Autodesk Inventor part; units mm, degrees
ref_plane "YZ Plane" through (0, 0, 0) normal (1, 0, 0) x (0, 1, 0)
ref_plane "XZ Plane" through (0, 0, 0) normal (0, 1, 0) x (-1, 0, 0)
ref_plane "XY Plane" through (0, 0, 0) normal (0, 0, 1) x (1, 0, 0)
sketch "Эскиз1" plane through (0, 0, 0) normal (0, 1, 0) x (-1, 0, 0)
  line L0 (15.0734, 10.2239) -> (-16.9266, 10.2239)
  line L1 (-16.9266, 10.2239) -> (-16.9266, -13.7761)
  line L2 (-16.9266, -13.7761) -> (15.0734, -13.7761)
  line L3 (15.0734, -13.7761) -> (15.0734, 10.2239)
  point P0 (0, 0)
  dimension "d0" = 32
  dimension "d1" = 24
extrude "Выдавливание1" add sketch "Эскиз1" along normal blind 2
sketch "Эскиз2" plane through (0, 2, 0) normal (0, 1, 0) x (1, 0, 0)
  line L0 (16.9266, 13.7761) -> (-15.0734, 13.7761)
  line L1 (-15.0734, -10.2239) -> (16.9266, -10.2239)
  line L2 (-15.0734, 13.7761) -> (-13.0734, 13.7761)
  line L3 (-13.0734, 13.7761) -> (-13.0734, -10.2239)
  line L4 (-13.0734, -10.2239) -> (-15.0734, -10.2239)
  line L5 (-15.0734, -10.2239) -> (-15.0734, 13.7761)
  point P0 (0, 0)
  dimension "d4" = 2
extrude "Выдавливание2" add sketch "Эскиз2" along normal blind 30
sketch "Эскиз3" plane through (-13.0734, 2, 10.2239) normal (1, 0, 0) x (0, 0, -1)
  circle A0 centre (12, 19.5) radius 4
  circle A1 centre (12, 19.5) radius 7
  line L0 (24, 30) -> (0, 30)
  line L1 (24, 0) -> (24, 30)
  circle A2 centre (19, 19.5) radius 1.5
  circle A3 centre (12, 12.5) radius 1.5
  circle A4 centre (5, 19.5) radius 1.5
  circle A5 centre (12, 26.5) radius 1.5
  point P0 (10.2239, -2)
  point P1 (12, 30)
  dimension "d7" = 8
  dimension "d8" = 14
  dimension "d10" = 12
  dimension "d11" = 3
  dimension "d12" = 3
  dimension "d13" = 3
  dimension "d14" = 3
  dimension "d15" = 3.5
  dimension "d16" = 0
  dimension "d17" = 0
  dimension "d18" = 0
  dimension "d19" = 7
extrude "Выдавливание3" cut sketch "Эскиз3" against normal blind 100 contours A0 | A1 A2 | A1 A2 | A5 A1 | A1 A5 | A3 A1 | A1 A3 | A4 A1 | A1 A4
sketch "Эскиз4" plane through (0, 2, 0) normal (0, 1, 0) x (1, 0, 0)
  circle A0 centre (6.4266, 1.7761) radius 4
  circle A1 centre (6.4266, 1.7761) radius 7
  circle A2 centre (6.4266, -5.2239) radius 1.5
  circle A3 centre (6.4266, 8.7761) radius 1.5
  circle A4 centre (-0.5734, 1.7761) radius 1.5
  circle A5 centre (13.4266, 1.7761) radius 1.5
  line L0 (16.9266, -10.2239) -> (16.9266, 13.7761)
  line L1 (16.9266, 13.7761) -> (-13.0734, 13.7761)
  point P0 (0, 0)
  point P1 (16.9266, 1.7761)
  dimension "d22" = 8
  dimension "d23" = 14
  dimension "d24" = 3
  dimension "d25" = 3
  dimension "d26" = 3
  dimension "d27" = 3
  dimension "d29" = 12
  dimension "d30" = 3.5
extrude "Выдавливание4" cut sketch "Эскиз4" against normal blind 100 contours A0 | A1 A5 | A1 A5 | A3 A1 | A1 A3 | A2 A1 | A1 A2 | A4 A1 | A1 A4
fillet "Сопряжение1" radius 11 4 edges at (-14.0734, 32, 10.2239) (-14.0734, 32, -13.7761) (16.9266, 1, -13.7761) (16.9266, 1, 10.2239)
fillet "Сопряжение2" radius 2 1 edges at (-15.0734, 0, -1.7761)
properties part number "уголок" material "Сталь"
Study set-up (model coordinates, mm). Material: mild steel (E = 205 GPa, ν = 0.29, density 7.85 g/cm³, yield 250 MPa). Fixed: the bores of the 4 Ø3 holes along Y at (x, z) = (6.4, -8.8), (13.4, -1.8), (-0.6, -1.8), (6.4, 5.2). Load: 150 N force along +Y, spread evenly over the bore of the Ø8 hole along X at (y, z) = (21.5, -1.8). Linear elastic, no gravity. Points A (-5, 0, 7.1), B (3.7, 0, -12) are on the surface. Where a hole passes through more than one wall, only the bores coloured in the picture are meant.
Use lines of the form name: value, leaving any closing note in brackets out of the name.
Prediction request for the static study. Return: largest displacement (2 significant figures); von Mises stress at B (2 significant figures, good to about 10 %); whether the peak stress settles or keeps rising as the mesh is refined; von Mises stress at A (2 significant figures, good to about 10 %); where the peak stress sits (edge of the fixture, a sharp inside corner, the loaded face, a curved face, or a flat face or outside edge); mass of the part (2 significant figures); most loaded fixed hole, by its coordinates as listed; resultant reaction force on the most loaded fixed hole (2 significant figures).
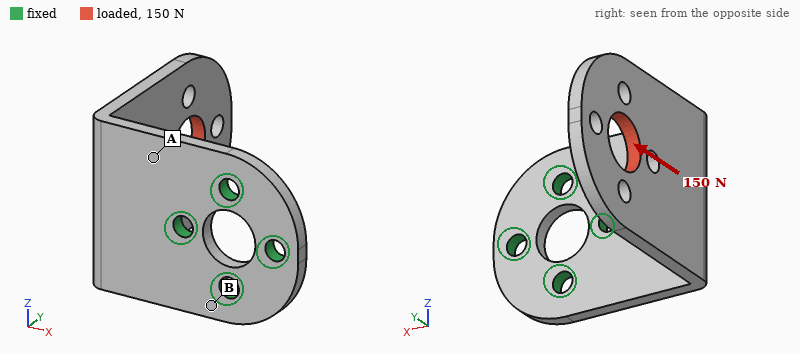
largest displacement: 0.14 mm
von Mises stress at B: 24 MPa
whether the peak stress settles or keeps rising as the mesh is refined: keeps rising
von Mises stress at A: 66 MPa
where the peak stress sits: edge of the fixture
mass of the part: 19 g
most loaded fixed hole, by its coordinates as listed: (-0.6, -1.8)
resultant reaction force on the most loaded fixed hole: 240 N
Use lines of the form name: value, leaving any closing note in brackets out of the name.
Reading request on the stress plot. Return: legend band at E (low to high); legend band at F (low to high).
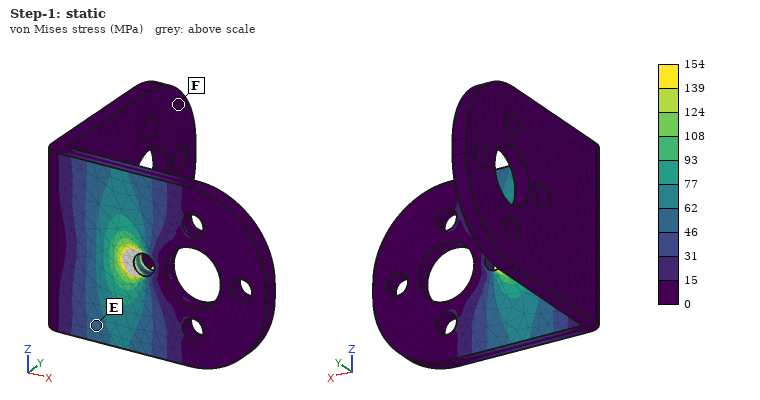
legend band at E: 46 to 62 MPa
legend band at F: 0 to 15 MPa
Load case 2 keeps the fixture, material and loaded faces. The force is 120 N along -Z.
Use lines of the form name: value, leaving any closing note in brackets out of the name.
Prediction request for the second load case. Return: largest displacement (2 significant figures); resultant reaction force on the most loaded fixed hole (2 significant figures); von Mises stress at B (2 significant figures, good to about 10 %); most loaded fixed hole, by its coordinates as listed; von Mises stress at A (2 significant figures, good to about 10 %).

largest displacement: 0.17 mm
resultant reaction force on the most loaded fixed hole: 140 N
von Mises stress at B: 88 MPa
most loaded fixed hole, by its coordinates as listed: (-0.6, -1.8)
von Mises stress at A: 80 MPa
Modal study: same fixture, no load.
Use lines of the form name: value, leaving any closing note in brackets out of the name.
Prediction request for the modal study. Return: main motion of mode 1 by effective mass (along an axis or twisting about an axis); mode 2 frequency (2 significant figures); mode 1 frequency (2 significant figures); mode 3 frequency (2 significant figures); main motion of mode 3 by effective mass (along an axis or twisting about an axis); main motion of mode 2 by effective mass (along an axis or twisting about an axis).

main motion of mode 1 by effective mass: along X
mode 2 frequency: 1900 Hz
mode 1 frequency: 1200 Hz
mode 3 frequency: 4100 Hz
main motion of mode 3 by effective mass: along Y
main motion of mode 2 by effective mass: along Z
